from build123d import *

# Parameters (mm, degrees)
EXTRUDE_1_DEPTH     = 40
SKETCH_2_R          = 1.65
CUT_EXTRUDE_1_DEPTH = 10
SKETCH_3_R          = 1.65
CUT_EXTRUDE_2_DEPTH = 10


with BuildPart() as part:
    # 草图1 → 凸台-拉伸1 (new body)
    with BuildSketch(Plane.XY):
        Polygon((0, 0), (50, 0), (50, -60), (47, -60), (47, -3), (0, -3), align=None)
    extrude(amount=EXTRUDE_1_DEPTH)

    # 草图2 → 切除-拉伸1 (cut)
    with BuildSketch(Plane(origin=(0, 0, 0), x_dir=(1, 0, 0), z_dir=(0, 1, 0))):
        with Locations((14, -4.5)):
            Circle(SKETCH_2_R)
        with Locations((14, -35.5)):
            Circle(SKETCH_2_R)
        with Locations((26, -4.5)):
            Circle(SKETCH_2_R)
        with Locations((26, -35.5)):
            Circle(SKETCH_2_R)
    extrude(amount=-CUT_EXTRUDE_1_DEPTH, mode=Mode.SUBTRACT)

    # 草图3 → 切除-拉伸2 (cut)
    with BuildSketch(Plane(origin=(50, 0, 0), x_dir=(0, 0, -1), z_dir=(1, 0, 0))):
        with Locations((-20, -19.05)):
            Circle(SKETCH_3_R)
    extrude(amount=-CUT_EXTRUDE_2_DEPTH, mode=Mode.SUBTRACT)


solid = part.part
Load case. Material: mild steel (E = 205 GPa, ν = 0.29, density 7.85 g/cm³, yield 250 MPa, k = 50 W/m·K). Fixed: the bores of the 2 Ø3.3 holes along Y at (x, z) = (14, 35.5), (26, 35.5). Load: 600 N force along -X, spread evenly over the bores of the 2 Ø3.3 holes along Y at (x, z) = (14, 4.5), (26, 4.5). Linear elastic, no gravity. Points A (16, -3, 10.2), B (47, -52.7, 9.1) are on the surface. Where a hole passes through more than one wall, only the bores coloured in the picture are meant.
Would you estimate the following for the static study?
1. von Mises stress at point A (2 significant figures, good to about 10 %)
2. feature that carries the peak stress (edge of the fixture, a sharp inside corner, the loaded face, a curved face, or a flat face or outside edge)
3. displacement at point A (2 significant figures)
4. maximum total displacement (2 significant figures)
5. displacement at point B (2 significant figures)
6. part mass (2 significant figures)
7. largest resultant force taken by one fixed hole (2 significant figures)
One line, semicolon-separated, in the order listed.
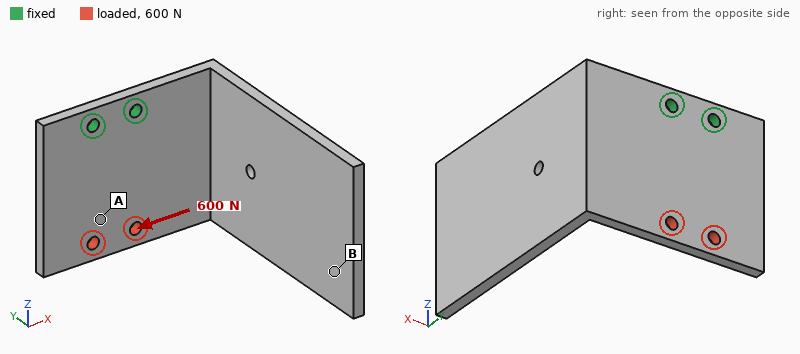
13 MPa; edge of the fixture; 9.5 µm; 17 µm; 13 µm; 100 g; 1.3 kN
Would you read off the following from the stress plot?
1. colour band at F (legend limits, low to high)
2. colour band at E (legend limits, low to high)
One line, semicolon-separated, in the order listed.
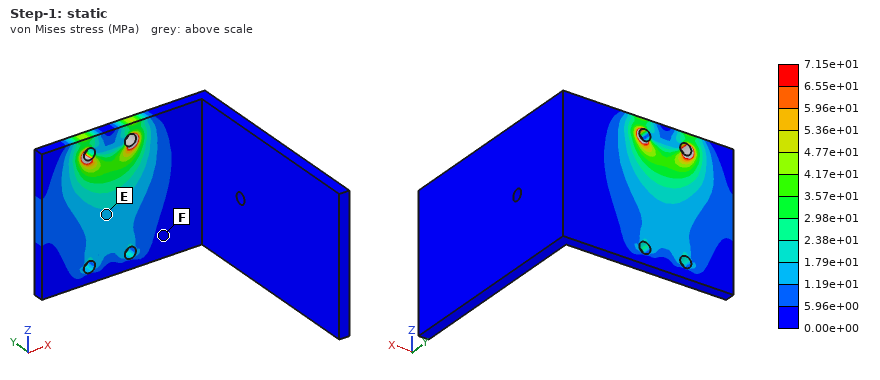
0.00e+00 to 5.96e+00 MPa; 1.19e+01 to 1.79e+01 MPa
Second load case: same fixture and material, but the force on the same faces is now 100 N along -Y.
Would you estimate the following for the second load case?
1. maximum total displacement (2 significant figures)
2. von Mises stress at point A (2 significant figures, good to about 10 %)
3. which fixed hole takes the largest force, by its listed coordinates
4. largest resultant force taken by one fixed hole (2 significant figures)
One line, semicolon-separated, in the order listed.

0.10 mm; 9.2 MPa; (26, 35.5); 54 N
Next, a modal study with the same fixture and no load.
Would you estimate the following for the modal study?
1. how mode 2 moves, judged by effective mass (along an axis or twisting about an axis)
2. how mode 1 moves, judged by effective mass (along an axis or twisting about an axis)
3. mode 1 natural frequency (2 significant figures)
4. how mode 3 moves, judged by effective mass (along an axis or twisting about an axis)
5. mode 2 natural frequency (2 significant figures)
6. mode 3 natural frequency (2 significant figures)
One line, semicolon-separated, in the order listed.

along Z; along X; 400 Hz; along Y; 560 Hz; 1600 Hz
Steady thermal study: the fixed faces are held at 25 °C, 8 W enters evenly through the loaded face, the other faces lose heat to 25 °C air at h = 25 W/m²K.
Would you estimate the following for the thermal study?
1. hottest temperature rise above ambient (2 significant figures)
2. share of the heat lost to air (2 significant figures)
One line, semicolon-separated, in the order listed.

41 K; 34 %
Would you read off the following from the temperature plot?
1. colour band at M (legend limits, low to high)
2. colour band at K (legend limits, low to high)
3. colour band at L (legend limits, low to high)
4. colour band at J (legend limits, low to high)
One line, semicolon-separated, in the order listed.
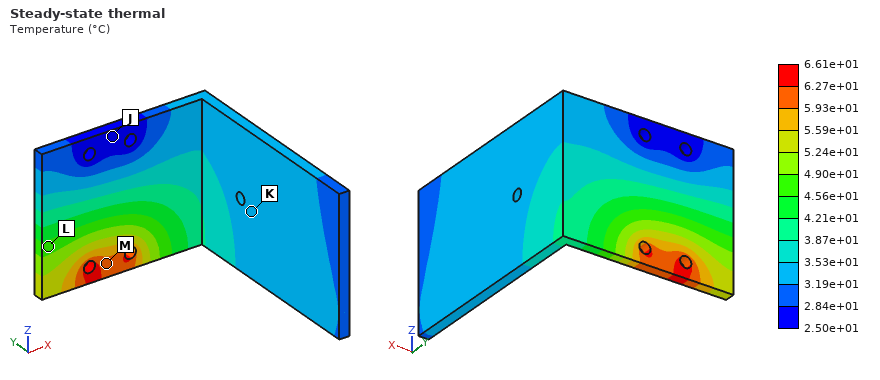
5.93e+01 to 6.27e+01 °C; 3.19e+01 to 3.53e+01 °C; 4.56e+01 to 4.90e+01 °C; 2.50e+01 to 2.84e+01 °C
